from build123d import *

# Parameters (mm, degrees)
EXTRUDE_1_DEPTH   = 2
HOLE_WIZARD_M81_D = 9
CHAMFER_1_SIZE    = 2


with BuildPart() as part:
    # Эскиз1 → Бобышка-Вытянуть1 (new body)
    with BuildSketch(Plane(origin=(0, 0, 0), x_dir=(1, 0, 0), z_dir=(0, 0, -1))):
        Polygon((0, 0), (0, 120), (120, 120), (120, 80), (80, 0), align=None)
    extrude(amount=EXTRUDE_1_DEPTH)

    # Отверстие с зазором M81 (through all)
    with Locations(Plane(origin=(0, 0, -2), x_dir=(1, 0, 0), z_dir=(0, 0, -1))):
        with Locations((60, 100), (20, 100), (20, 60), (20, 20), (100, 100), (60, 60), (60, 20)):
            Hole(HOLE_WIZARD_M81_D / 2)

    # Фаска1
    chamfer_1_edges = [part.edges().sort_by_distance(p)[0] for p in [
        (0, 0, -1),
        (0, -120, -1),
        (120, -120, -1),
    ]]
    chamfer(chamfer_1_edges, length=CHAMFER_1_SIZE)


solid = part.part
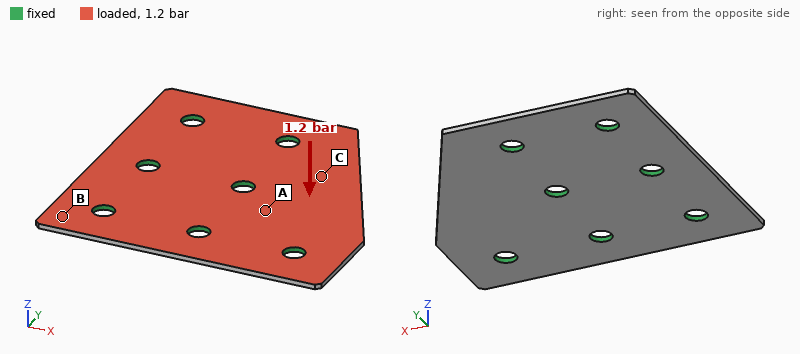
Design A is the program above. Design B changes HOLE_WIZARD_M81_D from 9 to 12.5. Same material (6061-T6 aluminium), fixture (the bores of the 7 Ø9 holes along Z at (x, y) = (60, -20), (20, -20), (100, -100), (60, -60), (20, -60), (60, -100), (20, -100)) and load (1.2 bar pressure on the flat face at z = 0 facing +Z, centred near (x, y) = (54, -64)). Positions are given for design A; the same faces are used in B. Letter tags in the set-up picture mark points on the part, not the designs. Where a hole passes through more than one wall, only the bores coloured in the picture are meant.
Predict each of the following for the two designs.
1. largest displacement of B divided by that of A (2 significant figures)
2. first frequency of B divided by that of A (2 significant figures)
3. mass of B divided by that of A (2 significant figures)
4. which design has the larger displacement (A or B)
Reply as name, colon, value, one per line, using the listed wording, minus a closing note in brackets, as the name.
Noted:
largest displacement of B divided by that of A: 0.83
first frequency of B divided by that of A: 1.1
mass of B divided by that of A: 0.97
which design has the larger displacement: A
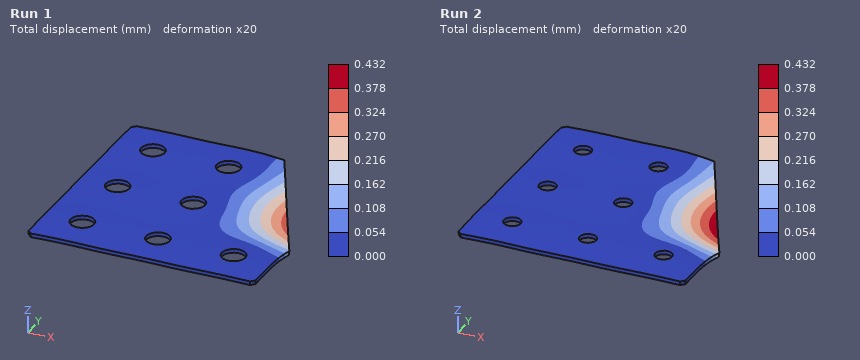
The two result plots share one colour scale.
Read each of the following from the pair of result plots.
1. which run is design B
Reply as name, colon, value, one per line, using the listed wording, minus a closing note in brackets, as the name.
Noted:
which run is design B: Run 1
